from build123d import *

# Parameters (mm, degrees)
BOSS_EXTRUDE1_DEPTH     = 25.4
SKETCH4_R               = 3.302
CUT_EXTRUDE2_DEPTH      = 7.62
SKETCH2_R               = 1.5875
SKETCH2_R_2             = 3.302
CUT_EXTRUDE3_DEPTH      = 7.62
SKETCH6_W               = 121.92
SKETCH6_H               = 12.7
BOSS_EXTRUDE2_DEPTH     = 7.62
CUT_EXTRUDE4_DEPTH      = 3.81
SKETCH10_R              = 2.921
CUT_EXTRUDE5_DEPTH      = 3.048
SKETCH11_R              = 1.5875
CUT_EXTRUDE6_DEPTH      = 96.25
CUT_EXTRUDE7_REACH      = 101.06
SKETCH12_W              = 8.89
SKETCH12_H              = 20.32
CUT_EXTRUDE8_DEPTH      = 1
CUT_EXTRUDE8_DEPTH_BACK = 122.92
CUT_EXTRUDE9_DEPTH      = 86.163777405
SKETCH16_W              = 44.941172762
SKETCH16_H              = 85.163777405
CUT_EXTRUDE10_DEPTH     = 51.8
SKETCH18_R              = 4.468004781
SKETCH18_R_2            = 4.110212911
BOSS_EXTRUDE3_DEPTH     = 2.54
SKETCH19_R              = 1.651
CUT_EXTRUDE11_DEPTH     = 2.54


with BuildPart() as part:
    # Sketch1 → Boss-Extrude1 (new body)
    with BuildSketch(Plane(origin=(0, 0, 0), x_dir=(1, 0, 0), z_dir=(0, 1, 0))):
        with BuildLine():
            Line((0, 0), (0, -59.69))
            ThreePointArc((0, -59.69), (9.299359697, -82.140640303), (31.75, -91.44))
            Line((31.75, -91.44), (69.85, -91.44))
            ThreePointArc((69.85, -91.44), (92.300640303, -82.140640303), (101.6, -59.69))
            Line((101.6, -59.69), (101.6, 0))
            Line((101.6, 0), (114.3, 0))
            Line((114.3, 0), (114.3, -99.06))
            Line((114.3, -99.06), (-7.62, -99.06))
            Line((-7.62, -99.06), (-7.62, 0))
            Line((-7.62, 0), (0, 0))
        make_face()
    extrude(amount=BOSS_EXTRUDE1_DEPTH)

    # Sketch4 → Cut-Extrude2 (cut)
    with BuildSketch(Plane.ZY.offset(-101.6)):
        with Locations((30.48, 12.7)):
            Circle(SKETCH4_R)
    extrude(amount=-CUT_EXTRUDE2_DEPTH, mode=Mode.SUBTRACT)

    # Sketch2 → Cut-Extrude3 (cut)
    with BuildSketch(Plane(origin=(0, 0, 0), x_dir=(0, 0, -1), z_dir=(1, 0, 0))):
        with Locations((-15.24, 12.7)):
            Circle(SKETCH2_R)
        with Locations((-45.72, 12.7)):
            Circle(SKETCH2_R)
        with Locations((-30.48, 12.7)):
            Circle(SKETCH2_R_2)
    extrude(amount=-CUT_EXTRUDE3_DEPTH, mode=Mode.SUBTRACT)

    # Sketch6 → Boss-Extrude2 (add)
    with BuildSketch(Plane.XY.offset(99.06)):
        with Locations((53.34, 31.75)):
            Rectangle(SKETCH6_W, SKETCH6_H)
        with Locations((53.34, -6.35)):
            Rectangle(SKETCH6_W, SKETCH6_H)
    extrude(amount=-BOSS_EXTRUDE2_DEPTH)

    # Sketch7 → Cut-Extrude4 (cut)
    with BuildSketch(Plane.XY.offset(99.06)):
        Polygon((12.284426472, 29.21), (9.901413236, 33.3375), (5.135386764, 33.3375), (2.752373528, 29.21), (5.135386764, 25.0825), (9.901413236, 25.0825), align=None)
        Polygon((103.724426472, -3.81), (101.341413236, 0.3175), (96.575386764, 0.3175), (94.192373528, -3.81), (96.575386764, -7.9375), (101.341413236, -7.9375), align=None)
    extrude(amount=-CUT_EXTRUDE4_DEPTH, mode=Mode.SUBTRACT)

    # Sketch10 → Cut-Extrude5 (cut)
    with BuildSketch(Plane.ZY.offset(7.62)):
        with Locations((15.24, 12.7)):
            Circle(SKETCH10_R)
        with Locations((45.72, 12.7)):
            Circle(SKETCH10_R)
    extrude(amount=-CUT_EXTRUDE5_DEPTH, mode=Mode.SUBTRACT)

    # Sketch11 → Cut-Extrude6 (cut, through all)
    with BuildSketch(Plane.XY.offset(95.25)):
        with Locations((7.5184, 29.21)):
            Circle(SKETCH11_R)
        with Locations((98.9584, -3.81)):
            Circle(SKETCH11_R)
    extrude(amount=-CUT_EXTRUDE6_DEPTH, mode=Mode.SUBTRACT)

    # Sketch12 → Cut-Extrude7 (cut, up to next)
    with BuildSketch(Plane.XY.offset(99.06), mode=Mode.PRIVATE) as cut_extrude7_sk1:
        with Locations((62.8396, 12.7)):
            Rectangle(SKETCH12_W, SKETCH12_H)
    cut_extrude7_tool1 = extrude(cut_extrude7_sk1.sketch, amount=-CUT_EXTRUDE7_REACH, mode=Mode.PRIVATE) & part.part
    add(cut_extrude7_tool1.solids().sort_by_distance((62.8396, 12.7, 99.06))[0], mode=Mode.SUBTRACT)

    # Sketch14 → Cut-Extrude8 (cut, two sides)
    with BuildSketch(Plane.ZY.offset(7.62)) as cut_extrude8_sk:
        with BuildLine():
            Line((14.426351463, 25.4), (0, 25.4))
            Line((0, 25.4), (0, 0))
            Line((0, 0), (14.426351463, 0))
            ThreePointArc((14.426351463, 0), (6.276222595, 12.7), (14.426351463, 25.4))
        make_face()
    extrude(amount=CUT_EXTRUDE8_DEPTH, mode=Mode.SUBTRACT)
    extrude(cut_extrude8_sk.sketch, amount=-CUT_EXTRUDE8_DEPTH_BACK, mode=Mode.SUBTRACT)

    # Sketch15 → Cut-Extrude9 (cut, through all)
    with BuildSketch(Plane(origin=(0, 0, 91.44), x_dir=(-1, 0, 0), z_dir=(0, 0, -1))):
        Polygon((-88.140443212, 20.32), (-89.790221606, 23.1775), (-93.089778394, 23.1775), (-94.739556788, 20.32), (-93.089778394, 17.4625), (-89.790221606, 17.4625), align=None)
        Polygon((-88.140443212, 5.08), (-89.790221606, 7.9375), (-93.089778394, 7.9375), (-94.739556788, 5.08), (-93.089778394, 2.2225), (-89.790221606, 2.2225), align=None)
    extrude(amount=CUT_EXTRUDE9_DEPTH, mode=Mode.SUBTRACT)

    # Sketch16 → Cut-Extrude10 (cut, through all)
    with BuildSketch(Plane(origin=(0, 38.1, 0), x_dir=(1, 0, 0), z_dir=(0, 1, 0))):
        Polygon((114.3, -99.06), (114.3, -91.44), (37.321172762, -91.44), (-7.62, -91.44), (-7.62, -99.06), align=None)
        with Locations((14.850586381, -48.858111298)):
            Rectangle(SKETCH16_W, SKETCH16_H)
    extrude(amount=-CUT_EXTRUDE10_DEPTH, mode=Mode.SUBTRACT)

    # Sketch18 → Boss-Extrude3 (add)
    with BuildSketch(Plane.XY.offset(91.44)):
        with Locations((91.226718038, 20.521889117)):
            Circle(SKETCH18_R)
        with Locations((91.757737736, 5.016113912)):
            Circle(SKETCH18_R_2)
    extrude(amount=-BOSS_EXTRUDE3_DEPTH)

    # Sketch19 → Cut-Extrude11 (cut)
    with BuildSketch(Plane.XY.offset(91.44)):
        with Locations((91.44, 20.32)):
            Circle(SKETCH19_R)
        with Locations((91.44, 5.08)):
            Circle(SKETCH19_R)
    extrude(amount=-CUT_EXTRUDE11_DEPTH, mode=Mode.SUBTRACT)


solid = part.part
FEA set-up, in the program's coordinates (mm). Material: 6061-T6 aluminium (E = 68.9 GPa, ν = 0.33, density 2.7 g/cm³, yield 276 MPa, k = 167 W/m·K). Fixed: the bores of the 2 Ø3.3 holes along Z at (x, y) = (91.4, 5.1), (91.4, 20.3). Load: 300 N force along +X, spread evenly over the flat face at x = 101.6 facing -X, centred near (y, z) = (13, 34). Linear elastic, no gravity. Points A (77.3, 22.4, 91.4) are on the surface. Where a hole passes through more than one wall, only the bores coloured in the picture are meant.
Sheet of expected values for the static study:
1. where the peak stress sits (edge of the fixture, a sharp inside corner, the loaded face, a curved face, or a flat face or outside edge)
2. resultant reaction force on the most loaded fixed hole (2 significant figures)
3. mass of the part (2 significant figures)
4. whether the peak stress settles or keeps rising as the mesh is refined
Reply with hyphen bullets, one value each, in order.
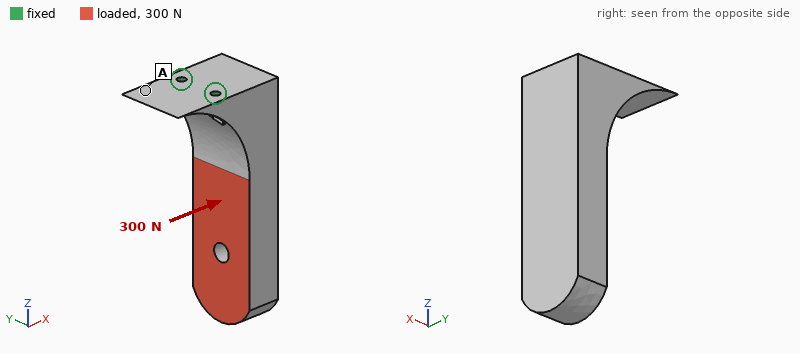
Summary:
- edge of the fixture
- 160 N
- 85 g
- keeps rising
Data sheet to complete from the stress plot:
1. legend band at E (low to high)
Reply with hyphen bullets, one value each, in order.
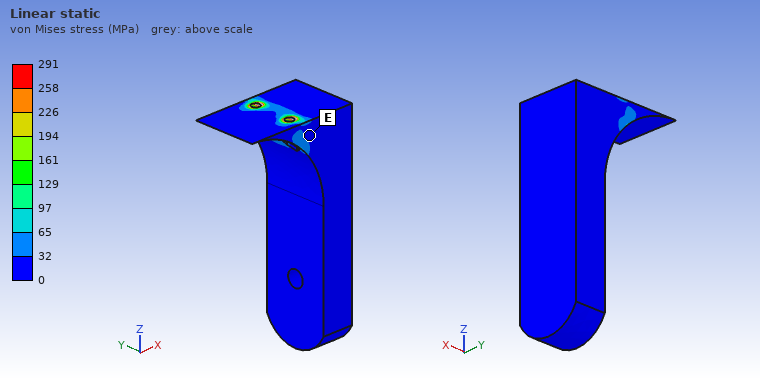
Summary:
- 0 to 32 MPa
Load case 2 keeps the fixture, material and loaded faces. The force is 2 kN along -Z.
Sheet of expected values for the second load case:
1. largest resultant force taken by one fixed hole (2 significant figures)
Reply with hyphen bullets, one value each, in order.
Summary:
- 1.0 kN
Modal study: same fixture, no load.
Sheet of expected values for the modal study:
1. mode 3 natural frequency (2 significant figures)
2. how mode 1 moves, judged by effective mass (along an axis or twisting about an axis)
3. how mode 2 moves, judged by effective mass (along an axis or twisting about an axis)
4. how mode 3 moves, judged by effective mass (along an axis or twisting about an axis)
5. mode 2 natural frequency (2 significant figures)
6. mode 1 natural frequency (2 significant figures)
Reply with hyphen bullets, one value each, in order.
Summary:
- 4900 Hz
- along X
- along Y
- along Z
- 1600 Hz
- 570 Hz
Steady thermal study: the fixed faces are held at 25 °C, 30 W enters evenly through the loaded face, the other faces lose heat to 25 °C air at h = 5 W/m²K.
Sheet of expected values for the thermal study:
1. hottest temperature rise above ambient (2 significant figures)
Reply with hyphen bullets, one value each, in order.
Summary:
- 39 K
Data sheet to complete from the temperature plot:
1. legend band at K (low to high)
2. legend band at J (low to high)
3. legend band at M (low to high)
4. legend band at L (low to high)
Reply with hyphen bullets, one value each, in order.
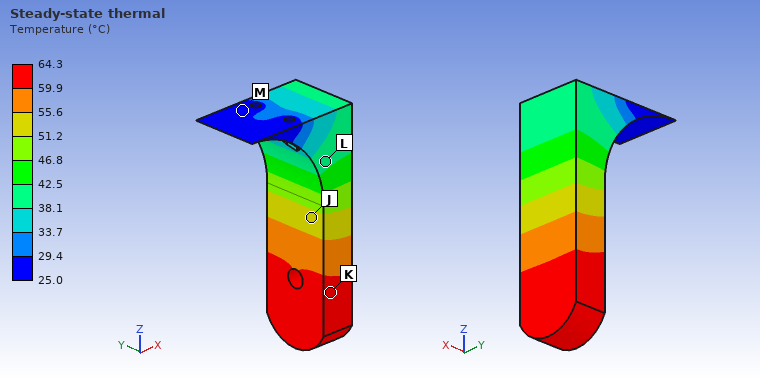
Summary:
- 59.9 to 64.3 °C
- 51.2 to 55.6 °C
- 25.0 to 29.4 °C
- 38.1 to 42.5 °C
